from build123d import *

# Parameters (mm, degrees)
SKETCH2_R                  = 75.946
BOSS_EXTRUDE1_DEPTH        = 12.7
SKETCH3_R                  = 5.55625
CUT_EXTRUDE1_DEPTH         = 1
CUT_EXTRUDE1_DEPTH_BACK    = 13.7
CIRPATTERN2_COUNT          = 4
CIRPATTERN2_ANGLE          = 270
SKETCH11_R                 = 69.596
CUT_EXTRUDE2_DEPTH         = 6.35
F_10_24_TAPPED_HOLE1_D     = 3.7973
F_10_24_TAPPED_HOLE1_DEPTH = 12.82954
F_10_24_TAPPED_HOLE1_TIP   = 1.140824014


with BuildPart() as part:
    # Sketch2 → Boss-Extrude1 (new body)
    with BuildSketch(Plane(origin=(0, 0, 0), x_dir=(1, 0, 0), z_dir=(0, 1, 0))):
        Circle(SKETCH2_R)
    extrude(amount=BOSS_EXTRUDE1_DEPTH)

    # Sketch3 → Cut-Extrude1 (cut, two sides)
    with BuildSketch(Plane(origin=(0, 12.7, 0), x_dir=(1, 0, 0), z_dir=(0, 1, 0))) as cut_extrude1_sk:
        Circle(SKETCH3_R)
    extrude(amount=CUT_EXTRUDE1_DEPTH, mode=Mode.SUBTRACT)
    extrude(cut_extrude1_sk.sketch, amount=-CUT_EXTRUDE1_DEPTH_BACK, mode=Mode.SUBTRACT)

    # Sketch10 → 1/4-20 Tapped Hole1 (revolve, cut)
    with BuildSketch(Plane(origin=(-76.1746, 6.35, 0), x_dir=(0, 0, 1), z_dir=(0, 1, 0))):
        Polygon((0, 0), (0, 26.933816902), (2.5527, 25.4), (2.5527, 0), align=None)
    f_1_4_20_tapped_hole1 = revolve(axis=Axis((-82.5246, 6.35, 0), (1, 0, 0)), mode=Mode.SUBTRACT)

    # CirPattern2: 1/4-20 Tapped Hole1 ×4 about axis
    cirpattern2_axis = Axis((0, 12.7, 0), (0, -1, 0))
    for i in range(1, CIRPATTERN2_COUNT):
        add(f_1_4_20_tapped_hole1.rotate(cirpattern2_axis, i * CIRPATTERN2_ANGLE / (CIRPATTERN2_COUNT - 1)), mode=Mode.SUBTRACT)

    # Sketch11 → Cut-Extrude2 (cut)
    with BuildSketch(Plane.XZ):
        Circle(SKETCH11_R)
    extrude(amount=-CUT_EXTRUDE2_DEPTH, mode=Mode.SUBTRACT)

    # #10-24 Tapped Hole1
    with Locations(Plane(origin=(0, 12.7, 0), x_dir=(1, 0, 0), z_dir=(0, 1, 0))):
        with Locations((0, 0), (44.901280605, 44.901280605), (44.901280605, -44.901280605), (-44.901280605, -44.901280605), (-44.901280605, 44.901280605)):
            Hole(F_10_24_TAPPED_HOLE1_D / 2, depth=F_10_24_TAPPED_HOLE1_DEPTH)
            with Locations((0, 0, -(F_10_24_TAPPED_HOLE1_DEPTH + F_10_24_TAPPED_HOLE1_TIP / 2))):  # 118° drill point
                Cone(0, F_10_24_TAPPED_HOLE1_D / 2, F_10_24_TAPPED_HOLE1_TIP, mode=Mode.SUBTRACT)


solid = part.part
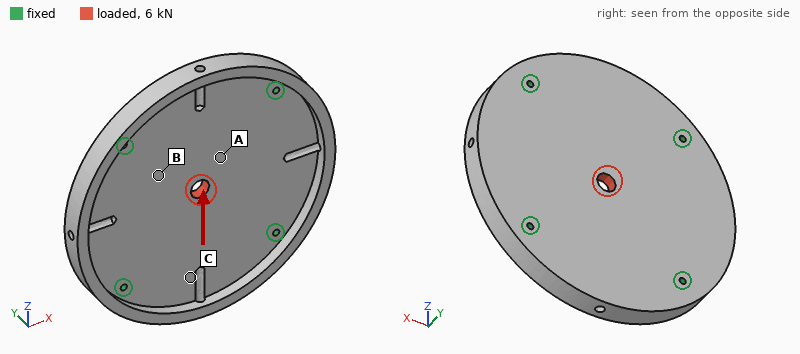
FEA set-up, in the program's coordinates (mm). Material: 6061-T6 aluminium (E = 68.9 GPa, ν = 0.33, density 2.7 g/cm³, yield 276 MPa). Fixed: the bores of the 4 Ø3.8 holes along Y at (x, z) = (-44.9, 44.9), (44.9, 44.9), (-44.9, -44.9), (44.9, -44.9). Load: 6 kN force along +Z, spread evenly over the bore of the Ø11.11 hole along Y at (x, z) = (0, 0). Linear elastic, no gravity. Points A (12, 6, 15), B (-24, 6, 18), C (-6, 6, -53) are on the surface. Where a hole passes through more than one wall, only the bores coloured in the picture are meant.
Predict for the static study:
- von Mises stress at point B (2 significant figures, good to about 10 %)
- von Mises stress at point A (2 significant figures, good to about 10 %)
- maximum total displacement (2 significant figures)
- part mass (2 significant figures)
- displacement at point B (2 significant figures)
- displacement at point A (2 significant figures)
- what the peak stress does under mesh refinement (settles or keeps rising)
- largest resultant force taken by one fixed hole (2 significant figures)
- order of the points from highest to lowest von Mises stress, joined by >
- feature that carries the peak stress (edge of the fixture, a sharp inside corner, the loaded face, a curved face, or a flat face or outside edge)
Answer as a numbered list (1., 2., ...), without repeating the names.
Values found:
1. 8.2 MPa
2. 12 MPa
3. 13 µm
4. 350 g
5. 5.3 µm
6. 7.8 µm
7. keeps rising
8. 1.5 kN
9. A > B > C
10. edge of the fixture
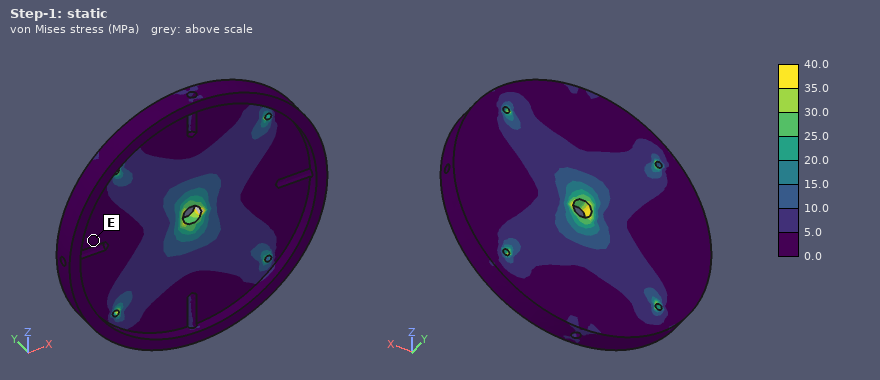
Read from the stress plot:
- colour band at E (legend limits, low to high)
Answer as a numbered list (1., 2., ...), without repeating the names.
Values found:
1. 0.0 to 5.0 MPa
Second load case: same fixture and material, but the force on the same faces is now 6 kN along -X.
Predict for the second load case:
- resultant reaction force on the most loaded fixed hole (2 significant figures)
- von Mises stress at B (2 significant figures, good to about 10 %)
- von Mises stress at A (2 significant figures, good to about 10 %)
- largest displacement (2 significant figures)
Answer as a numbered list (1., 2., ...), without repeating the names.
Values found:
1. 1.5 kN
2. 8.8 MPa
3. 11 MPa
4. 13 µm
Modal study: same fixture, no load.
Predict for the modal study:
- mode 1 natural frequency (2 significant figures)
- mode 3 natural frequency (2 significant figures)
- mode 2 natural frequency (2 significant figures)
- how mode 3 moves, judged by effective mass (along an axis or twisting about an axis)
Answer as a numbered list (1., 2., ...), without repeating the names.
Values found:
1. 2700 Hz
2. 3400 Hz
3. 2700 Hz
4. twisting about X
